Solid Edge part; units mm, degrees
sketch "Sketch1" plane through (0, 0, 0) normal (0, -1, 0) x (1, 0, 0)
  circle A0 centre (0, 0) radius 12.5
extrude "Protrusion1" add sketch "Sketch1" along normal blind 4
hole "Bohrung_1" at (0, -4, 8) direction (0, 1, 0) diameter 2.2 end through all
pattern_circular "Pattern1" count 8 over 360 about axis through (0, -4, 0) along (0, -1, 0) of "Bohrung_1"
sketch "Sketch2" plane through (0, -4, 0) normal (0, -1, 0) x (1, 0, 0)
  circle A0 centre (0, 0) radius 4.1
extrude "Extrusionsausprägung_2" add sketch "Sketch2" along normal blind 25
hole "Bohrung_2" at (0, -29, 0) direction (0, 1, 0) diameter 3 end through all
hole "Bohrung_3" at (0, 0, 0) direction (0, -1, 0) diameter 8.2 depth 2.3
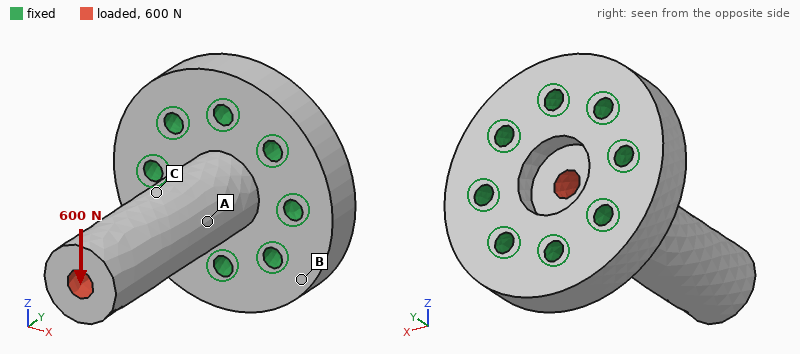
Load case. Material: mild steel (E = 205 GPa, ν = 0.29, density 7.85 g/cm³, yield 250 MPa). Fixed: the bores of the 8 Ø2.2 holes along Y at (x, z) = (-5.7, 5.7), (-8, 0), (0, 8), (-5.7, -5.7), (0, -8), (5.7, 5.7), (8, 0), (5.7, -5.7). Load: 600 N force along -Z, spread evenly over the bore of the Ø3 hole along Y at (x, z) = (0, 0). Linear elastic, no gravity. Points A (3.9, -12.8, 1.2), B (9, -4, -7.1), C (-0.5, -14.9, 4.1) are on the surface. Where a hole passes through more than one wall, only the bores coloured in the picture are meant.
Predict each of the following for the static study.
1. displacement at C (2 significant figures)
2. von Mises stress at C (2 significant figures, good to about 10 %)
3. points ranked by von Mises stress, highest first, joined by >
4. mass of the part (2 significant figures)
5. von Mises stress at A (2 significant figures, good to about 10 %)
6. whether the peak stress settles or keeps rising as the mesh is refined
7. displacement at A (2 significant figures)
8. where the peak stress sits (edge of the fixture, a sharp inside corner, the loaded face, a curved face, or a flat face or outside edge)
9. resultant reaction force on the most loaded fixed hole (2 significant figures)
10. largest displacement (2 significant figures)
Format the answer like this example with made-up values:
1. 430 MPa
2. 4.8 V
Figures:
1. 17 µm
2. 41 MPa
3. C > A > B
4. 22 g
5. 25 MPa
6. keeps rising
7. 12 µm
8. a sharp inside corner
9. 390 N
10. 43 µm
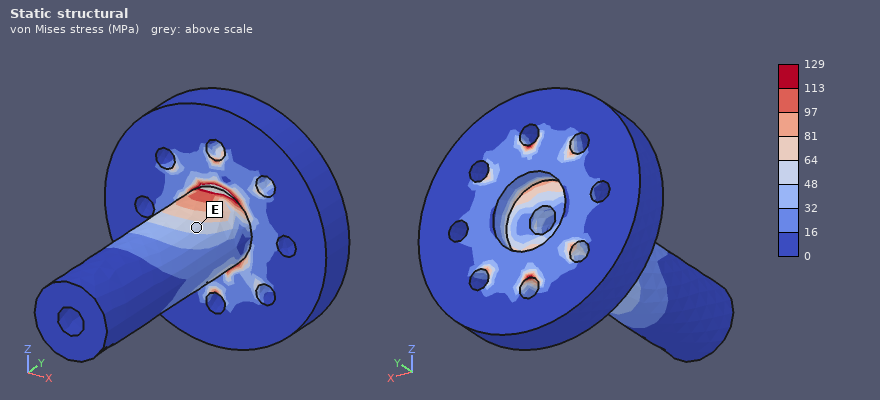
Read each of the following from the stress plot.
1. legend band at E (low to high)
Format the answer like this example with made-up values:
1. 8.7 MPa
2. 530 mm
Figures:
1. 48 to 64 MPa
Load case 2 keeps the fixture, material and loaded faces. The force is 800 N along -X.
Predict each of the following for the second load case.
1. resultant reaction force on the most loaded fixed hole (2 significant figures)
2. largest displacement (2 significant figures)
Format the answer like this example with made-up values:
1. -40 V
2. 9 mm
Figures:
1. 520 N
2. 57 µm
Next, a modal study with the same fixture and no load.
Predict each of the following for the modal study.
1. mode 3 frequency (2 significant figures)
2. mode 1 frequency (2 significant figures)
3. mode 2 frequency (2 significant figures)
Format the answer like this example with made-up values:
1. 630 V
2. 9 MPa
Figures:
1. 30 kHz
2. 7500 Hz
3. 7500 Hz
